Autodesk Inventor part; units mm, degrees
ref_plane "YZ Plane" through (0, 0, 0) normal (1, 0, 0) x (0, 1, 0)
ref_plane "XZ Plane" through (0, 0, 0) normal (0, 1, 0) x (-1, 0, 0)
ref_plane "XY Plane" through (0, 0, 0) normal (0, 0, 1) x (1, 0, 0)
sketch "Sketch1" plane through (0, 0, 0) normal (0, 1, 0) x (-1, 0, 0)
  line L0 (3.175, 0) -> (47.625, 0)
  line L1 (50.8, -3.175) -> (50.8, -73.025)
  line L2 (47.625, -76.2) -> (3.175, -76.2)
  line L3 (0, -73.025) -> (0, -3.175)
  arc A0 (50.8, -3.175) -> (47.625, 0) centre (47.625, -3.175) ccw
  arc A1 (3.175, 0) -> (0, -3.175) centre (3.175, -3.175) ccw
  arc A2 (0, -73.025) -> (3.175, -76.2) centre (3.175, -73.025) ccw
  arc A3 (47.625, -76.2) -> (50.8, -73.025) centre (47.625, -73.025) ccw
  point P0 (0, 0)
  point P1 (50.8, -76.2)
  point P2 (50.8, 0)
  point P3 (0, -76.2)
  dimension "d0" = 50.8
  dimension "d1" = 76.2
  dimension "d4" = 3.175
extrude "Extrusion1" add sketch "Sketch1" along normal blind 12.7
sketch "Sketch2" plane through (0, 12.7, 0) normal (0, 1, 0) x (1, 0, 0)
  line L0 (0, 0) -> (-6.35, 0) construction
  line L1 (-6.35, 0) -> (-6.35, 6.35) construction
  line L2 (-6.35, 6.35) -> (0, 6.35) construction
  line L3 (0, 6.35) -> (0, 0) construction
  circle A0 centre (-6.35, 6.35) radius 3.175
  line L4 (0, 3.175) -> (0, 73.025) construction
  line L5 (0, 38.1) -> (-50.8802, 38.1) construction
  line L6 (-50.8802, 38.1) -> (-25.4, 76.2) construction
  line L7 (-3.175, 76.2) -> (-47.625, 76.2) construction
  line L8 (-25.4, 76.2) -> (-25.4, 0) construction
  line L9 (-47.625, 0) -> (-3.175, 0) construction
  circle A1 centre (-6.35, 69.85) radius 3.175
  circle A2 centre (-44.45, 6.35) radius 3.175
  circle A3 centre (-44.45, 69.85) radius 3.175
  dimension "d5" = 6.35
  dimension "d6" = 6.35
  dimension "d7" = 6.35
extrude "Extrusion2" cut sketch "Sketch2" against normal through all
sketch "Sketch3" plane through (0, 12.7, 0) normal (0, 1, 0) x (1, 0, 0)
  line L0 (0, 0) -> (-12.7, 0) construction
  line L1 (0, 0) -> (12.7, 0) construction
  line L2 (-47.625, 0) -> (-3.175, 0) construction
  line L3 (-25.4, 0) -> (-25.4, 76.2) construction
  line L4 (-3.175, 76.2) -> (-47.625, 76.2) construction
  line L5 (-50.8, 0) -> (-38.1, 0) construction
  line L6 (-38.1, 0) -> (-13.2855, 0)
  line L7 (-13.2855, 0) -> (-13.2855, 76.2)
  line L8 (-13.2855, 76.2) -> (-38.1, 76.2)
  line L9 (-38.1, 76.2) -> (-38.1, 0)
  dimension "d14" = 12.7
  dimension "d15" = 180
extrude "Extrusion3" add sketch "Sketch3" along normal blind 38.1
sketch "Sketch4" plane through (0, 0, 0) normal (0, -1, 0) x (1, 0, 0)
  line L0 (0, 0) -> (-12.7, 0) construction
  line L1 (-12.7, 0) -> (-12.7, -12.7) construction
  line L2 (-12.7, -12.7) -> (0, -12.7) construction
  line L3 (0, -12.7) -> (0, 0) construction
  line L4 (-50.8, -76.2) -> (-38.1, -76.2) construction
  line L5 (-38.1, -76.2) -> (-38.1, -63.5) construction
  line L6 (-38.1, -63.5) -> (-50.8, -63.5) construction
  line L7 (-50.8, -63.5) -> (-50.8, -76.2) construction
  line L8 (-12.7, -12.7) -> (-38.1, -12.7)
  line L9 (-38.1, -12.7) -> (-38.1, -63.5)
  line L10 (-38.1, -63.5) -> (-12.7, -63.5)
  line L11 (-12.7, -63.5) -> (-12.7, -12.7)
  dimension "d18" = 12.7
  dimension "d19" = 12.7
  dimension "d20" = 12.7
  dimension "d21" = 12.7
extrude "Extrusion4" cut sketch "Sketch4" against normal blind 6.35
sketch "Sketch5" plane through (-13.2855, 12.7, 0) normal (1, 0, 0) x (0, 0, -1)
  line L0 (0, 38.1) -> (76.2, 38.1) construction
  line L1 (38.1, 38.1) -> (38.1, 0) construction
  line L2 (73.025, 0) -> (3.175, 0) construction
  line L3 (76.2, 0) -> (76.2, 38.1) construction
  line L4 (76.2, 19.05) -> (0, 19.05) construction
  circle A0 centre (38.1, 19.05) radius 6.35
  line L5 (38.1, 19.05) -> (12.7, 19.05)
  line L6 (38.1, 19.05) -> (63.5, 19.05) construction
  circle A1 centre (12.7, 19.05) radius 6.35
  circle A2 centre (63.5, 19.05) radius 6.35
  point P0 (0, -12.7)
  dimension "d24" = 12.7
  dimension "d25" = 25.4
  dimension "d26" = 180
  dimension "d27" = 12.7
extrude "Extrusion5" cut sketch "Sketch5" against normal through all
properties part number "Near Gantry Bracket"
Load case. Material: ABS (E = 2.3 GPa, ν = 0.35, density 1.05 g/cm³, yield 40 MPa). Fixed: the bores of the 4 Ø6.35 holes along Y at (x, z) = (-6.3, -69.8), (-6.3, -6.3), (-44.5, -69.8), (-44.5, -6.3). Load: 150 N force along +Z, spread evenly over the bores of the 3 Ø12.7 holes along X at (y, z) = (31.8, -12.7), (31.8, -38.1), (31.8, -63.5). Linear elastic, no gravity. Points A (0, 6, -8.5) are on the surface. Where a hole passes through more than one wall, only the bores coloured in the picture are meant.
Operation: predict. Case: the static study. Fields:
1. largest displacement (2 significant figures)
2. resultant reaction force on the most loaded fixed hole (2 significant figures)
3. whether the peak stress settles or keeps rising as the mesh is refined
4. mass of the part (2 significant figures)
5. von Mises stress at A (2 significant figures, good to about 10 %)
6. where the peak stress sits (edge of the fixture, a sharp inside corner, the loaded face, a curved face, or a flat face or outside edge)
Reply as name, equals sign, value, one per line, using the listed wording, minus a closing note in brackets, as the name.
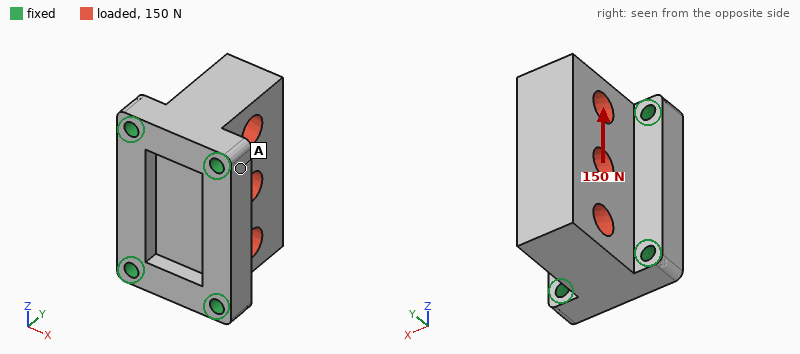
largest displacement = 8.9 µm
resultant reaction force on the most loaded fixed hole = 52 N
whether the peak stress settles or keeps rising as the mesh is refined = keeps rising
mass of the part = 110 g
von Mises stress at A = 0.085 MPa
where the peak stress sits = edge of the fixture
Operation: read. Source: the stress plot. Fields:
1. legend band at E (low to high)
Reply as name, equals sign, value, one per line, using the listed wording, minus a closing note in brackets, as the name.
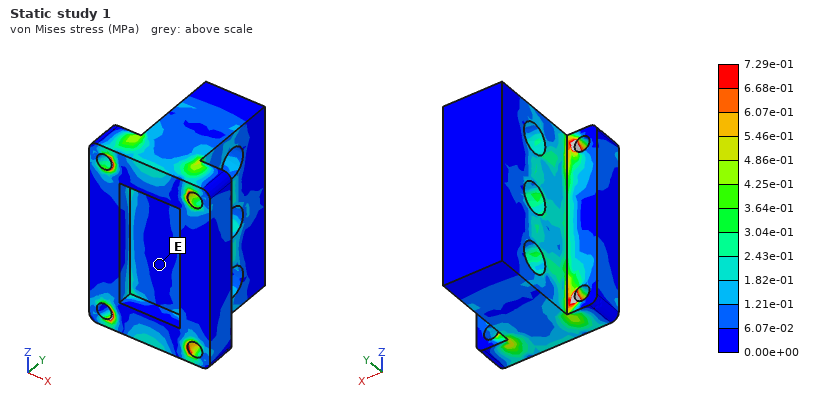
legend band at E = 0.00e+00 to 6.07e-02 MPa
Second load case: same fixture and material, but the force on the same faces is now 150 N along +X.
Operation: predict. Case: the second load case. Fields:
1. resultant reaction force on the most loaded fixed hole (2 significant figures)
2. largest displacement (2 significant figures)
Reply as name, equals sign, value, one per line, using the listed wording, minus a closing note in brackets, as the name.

resultant reaction force on the most loaded fixed hole = 70 N
largest displacement = 22 µm
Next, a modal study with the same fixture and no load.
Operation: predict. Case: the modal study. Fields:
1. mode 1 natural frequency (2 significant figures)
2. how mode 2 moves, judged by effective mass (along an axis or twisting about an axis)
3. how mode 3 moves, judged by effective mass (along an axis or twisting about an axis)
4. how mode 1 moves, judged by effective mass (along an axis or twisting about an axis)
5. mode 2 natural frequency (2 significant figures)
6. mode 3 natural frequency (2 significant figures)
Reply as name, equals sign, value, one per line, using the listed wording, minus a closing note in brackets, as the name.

mode 1 natural frequency = 1800 Hz
how mode 2 moves, judged by effective mass = along Z
how mode 3 moves, judged by effective mass = twisting about Y
how mode 1 moves, judged by effective mass = along X
mode 2 natural frequency = 2800 Hz
mode 3 natural frequency = 3200 Hz
